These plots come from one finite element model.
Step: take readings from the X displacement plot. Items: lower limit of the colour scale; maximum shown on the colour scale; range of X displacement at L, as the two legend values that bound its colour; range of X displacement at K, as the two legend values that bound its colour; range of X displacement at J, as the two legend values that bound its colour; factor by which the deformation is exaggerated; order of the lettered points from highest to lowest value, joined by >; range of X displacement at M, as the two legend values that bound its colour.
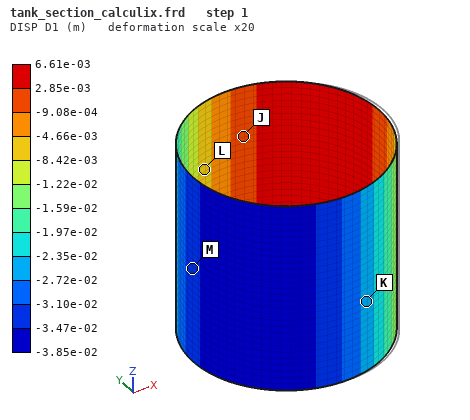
-3.85e-02 m
6.61e-03 m
-8.42e-03 to -4.66e-03 m
-2.72e-02 to -2.35e-02 m
-9.08e-04 to 2.85e-03 m
20
J > L > K > M
-3.47e-02 to -3.10e-02 m
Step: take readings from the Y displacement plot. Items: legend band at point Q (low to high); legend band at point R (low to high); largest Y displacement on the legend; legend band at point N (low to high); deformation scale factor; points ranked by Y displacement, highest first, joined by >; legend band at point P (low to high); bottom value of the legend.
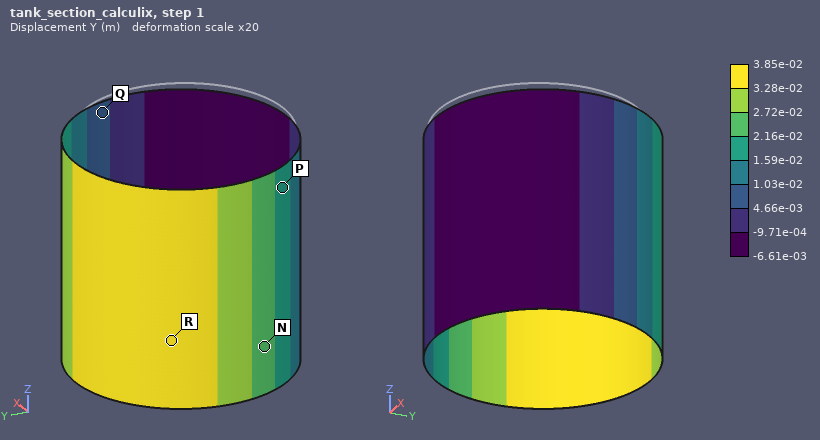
4.66e-03 to 1.03e-02 m
3.28e-02 to 3.85e-02 m
3.85e-02 m
2.16e-02 to 2.72e-02 m
20
R > N > P > Q
1.59e-02 to 2.16e-02 m
-6.61e-03 m
